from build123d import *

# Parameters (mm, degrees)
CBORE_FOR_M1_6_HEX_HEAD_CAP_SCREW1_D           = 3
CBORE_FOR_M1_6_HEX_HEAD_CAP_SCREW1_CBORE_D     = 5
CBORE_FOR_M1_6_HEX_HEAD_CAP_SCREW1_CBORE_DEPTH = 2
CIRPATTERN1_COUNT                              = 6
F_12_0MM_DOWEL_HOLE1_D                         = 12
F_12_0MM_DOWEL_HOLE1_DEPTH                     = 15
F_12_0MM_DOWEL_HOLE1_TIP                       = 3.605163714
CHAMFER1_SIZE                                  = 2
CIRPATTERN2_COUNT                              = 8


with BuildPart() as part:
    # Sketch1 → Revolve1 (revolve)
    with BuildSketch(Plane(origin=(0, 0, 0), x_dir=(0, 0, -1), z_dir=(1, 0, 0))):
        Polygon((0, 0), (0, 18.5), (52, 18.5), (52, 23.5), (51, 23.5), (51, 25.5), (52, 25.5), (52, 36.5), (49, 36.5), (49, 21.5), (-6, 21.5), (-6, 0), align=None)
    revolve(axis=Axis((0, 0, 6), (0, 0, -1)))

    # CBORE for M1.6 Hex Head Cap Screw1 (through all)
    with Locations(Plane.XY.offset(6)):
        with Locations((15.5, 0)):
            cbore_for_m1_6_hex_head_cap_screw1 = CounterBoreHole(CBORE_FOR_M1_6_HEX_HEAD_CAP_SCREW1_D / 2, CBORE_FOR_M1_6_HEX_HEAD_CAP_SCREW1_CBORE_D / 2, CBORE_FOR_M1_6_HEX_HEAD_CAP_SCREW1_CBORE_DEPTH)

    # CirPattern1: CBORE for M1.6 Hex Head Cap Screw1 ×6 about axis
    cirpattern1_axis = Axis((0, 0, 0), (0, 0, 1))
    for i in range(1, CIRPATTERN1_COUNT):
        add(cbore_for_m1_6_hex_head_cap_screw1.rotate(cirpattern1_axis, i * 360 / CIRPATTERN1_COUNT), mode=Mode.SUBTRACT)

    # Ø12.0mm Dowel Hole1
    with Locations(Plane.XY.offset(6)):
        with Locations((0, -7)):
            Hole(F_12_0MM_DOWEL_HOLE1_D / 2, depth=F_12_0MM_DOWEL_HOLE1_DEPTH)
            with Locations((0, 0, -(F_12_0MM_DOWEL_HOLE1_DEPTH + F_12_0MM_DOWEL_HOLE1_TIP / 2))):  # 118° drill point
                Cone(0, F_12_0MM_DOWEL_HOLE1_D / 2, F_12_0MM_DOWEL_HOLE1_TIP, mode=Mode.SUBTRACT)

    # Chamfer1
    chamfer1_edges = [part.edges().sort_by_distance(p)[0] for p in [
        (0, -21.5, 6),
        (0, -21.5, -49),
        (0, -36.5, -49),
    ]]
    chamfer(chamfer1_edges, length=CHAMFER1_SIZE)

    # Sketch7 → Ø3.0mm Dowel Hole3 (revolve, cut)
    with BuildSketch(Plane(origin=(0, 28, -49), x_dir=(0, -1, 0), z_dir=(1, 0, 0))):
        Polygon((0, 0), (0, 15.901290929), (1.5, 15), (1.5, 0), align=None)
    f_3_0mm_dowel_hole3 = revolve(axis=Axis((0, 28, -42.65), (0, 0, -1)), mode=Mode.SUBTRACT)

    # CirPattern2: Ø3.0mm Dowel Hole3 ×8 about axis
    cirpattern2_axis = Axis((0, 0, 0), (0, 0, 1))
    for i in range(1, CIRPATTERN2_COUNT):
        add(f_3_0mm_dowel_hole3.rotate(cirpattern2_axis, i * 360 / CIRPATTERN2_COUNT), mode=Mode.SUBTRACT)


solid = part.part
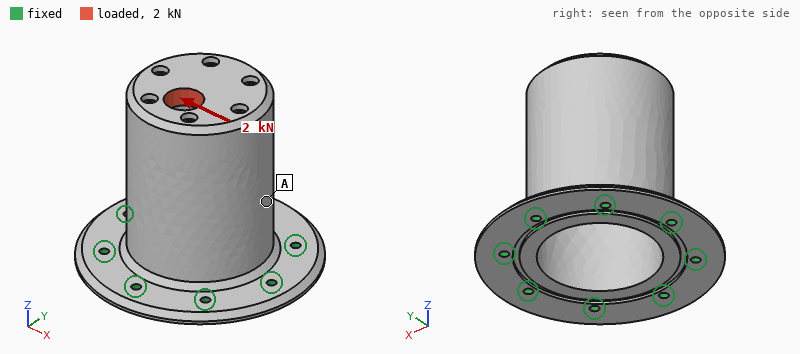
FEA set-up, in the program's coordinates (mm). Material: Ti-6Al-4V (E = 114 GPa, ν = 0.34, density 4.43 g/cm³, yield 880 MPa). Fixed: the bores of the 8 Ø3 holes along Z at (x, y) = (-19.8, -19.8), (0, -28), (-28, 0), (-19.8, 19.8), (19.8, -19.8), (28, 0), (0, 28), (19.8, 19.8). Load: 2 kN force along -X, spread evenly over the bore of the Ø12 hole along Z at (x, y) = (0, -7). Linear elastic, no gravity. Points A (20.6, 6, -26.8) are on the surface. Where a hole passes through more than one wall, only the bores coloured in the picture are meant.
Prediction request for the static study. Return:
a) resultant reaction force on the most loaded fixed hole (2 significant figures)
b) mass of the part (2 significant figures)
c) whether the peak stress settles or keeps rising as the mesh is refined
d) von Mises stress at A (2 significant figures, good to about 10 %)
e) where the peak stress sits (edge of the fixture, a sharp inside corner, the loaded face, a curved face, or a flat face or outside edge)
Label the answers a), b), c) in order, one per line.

a) 1.2 kN
b) 150 g
c) keeps rising
d) 14 MPa
e) edge of the fixture
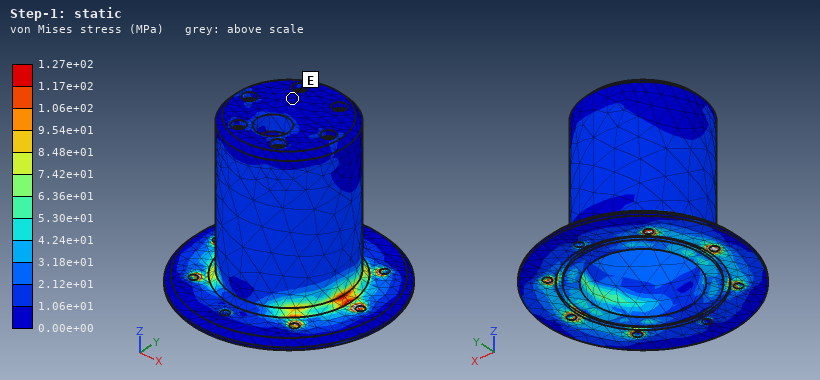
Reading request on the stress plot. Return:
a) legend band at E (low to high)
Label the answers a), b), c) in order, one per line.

a) 0.00e+00 to 1.06e+01 MPa
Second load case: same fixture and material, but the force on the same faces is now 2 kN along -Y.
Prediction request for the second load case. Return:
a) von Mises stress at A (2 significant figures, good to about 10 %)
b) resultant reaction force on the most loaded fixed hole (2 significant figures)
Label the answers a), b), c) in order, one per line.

a) 18 MPa
b) 1.2 kN
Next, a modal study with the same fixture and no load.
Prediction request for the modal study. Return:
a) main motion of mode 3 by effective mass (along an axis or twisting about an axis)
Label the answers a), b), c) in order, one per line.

a) along Z
